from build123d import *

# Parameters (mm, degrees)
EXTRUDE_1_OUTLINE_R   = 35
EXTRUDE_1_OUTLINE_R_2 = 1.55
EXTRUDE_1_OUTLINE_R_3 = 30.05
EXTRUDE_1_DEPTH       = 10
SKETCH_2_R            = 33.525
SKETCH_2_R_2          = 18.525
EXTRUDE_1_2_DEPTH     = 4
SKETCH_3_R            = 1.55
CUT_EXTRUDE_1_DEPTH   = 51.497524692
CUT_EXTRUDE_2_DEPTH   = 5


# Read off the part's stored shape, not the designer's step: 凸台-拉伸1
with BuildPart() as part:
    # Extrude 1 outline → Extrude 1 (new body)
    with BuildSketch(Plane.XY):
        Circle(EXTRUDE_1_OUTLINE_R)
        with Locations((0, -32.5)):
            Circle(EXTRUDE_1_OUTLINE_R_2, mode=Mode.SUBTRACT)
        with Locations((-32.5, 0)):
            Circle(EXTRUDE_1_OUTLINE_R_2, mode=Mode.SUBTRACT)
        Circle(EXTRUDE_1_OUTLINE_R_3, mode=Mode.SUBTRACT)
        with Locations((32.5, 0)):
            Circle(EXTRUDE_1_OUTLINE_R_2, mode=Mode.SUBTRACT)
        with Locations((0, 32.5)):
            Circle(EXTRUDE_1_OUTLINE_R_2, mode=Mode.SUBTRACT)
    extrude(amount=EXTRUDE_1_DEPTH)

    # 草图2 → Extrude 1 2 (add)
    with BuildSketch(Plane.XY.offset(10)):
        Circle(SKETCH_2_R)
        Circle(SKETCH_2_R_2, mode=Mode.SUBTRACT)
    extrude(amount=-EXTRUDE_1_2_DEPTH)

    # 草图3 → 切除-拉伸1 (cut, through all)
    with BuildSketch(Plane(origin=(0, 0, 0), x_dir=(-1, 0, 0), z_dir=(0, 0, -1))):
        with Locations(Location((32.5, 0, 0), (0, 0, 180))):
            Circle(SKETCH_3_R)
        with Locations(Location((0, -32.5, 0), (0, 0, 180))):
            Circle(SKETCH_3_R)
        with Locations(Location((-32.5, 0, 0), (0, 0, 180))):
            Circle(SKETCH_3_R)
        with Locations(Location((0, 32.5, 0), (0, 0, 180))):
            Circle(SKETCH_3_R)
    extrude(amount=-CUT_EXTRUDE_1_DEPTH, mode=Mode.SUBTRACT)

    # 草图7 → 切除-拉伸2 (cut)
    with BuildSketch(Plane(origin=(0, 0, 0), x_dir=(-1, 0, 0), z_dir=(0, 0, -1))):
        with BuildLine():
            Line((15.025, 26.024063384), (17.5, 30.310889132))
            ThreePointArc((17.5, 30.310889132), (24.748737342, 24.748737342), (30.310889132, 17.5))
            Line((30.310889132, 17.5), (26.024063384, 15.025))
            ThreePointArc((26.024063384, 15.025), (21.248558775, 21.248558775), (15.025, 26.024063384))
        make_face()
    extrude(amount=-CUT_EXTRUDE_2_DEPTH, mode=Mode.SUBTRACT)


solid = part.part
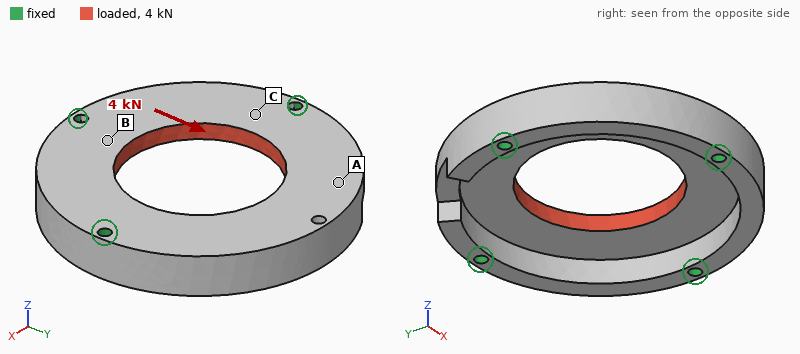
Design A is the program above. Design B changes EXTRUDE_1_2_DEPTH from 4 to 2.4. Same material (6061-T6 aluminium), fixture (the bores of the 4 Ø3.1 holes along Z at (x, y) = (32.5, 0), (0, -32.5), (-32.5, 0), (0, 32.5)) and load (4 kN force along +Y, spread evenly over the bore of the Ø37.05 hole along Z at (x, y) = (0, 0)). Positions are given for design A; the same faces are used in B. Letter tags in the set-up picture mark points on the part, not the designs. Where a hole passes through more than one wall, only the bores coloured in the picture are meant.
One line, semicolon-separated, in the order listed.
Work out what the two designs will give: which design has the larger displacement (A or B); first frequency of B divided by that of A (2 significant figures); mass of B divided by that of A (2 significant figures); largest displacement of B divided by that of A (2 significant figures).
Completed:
B; 0.92; 0.83; 1.5
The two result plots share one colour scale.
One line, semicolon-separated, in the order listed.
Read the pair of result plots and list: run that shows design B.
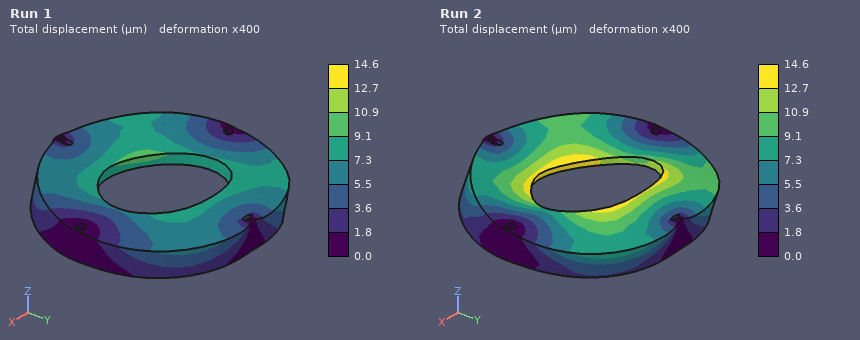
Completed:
Run 2
